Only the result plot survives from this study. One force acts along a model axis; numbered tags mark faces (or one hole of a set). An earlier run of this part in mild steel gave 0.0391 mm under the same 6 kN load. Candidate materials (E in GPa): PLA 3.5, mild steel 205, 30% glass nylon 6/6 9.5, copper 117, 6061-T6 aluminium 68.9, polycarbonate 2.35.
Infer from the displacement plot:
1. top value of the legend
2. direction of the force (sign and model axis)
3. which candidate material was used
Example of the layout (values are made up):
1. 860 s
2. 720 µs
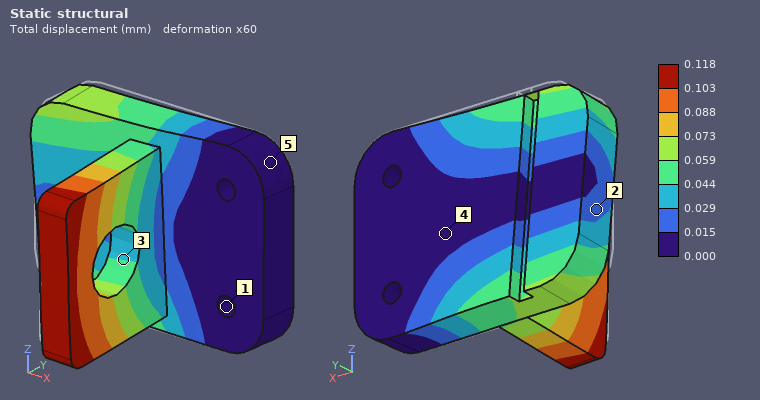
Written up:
1. 0.118 mm
2. -Z
3. 6061-T6 aluminium
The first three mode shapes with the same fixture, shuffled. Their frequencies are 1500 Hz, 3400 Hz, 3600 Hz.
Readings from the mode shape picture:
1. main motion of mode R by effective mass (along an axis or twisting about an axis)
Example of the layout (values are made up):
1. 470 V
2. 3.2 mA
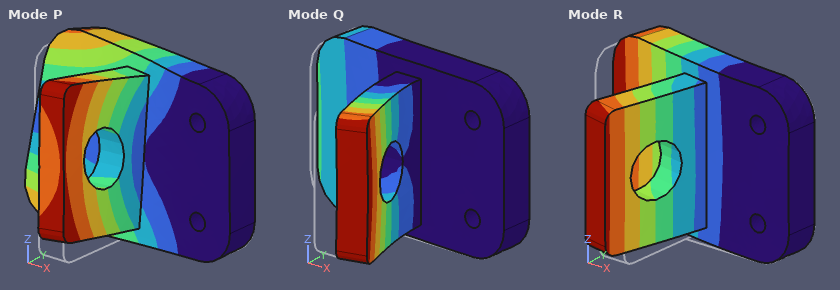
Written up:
1. along Y
